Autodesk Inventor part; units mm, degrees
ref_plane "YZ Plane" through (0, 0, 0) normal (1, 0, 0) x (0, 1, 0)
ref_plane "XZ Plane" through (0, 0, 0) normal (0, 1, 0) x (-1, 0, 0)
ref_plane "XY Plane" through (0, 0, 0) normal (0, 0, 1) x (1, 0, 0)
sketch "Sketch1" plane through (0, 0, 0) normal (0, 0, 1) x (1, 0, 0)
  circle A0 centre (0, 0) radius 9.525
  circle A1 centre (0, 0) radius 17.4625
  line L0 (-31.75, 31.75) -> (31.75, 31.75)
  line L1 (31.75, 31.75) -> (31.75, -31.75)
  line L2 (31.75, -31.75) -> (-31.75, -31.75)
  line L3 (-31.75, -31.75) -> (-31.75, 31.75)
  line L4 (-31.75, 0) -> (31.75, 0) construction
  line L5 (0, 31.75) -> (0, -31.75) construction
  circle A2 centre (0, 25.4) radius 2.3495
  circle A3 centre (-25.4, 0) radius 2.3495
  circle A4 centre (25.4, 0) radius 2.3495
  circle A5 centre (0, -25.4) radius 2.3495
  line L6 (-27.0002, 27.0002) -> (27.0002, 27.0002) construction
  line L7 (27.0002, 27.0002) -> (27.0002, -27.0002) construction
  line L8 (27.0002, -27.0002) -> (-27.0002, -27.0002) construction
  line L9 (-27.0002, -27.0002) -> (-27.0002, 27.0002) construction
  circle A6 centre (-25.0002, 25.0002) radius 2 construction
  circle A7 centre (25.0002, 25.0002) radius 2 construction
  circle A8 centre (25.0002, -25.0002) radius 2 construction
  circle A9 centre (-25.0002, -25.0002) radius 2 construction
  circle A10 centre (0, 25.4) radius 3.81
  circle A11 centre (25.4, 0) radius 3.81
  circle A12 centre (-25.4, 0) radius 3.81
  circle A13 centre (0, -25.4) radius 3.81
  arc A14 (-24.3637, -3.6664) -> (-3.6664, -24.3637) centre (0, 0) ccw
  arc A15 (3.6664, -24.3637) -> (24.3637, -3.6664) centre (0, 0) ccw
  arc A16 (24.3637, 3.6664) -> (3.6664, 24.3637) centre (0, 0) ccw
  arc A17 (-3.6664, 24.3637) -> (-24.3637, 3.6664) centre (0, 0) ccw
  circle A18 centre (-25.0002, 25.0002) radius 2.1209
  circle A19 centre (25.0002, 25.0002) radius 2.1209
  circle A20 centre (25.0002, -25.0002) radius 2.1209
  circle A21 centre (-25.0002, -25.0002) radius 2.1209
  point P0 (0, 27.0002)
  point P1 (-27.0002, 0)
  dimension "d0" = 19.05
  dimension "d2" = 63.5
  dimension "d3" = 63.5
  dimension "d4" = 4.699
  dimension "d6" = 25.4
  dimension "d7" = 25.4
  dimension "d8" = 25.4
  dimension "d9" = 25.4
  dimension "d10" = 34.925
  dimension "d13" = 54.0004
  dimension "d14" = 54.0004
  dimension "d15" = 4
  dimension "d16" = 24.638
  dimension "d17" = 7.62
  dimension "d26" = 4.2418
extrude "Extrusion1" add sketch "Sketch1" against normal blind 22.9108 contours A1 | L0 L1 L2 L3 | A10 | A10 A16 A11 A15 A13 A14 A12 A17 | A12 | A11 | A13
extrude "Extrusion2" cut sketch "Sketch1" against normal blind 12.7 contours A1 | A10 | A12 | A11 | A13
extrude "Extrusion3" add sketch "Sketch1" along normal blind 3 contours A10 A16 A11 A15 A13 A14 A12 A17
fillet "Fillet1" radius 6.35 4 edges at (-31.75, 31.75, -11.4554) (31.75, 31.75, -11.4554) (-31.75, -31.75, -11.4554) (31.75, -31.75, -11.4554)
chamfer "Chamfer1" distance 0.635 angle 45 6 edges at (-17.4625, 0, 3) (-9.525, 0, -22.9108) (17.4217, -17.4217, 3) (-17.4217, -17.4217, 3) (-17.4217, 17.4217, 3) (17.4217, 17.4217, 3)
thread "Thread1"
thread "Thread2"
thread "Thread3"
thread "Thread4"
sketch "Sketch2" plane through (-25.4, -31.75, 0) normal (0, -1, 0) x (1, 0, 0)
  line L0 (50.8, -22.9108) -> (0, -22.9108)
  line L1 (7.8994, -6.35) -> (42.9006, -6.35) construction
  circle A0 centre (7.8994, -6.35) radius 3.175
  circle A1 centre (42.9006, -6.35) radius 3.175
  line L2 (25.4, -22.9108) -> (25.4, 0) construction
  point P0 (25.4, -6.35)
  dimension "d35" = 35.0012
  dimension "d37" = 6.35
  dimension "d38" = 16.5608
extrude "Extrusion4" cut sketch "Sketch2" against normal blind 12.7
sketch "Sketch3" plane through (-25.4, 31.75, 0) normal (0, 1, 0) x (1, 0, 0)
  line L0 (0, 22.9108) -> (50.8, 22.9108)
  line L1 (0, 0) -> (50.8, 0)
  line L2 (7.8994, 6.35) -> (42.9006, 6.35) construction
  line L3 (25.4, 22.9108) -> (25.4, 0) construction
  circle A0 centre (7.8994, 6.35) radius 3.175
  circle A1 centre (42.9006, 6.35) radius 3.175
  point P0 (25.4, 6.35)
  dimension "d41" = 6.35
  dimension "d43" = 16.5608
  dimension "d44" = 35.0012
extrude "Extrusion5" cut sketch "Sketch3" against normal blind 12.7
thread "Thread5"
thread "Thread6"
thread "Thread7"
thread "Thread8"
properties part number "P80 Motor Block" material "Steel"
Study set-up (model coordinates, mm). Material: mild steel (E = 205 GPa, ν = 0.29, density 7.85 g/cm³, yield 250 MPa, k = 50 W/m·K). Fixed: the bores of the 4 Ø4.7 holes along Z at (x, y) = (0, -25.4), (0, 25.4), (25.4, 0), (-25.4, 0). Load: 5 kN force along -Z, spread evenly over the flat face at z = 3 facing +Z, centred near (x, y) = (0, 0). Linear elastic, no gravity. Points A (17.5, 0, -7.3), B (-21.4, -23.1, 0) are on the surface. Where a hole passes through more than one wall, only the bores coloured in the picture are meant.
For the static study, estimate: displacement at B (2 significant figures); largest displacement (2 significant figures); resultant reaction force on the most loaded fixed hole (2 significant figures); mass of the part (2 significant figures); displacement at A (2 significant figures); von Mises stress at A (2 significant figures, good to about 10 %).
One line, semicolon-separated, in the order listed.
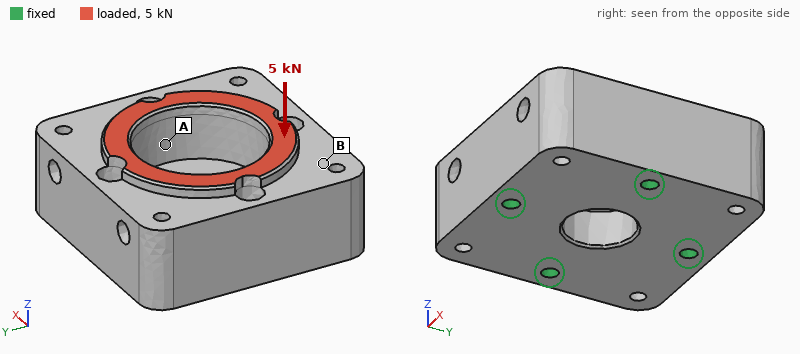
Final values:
0.50 µm; 0.85 µm; 1.3 kN; 570 g; 0.54 µm; 6.6 MPa
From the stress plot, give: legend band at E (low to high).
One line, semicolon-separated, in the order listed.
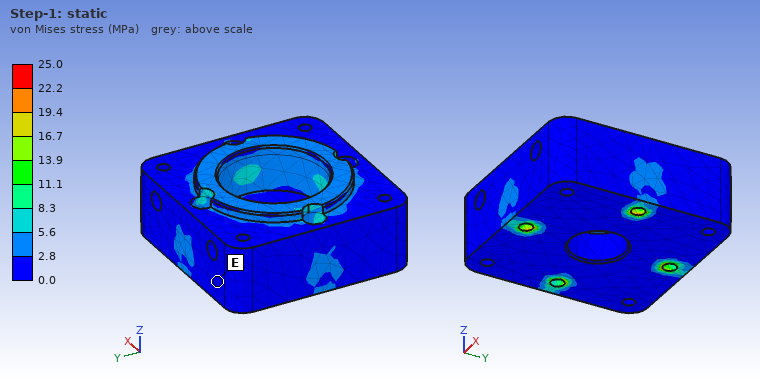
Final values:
0.0 to 2.8 MPa
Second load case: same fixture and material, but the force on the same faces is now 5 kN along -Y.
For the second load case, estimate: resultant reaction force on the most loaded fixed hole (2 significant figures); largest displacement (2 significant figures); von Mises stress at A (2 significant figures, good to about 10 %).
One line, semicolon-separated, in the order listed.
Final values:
2.0 kN; 3.4 µm; 15 MPa
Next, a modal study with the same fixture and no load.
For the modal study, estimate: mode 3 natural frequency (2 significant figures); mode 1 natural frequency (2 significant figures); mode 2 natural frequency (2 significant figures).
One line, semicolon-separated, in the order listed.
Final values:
15 kHz; 13 kHz; 15 kHz
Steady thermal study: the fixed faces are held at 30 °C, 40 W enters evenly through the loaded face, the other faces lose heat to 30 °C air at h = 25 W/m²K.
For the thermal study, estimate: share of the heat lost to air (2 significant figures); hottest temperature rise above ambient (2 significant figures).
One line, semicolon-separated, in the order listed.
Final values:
6.6 %; 15 K
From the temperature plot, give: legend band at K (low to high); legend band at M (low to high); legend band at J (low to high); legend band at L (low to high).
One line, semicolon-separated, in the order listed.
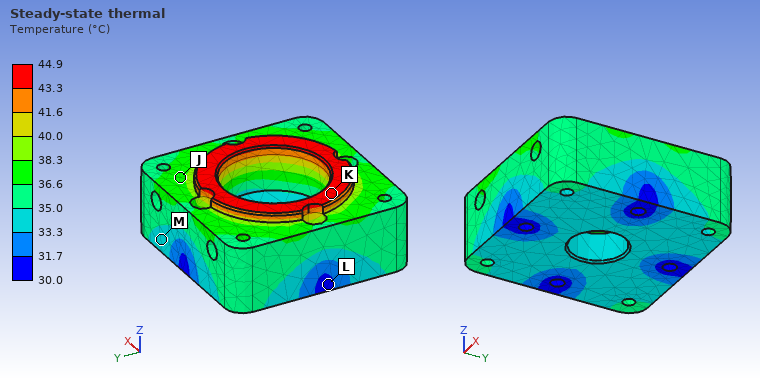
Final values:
43.3 to 44.9 °C; 33.3 to 35.0 °C; 36.6 to 38.3 °C; 30.0 to 31.7 °C
